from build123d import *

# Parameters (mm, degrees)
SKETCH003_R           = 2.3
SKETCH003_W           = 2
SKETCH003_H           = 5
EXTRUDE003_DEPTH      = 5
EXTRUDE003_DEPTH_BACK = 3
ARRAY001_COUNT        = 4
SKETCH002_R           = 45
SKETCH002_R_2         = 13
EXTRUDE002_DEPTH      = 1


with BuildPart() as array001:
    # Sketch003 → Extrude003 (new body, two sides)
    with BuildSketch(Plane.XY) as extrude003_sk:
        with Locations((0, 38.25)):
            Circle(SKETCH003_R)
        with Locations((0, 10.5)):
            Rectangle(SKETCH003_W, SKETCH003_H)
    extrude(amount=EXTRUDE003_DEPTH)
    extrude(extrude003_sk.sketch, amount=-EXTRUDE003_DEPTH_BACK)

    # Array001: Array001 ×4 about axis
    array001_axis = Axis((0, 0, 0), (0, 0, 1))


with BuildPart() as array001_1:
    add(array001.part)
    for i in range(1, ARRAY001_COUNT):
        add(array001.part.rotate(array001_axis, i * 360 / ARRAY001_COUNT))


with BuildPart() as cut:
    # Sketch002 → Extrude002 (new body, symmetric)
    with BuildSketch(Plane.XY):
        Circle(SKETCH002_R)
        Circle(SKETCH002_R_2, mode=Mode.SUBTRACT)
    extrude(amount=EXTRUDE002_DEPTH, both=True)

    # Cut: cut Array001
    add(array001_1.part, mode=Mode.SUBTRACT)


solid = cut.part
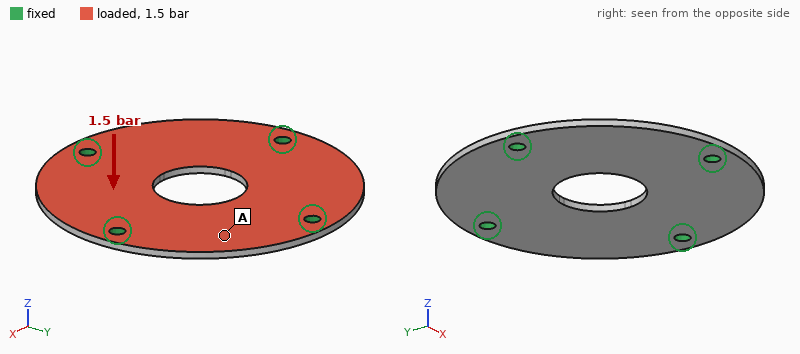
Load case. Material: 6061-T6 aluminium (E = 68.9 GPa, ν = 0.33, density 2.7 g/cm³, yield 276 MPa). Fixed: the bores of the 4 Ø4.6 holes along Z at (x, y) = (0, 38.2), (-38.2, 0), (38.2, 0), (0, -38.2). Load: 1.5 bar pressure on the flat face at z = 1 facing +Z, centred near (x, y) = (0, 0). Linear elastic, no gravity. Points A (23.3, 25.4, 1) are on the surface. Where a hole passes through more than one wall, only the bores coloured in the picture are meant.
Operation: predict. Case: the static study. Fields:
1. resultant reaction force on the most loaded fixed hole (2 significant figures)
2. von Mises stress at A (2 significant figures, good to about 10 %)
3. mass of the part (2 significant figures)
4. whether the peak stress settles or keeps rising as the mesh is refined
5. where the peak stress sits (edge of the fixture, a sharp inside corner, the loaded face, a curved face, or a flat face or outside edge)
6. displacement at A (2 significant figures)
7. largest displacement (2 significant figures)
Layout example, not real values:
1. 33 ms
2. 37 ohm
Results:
1. 220 N
2. 27 MPa
3. 31 g
4. keeps rising
5. edge of the fixture
6. 0.080 mm
7. 0.11 mm
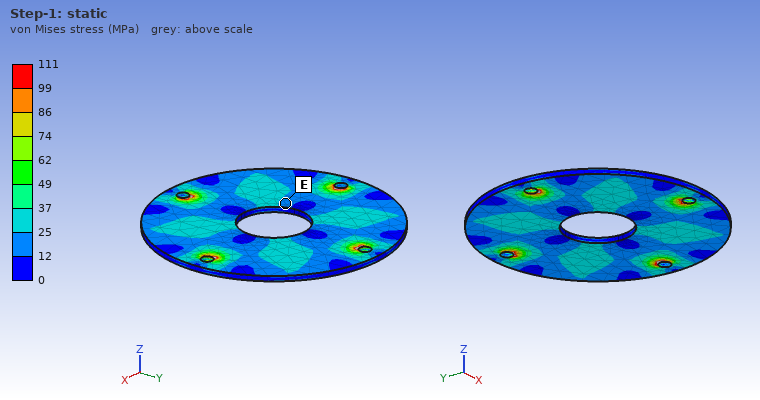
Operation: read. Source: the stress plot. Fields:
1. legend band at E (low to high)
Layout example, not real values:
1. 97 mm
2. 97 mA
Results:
1. 12 to 25 MPa
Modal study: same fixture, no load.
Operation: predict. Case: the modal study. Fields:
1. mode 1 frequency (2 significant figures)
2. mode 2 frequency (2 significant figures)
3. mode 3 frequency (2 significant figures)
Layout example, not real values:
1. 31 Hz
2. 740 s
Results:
1. 3000 Hz
2. 3000 Hz
3. 3100 Hz
